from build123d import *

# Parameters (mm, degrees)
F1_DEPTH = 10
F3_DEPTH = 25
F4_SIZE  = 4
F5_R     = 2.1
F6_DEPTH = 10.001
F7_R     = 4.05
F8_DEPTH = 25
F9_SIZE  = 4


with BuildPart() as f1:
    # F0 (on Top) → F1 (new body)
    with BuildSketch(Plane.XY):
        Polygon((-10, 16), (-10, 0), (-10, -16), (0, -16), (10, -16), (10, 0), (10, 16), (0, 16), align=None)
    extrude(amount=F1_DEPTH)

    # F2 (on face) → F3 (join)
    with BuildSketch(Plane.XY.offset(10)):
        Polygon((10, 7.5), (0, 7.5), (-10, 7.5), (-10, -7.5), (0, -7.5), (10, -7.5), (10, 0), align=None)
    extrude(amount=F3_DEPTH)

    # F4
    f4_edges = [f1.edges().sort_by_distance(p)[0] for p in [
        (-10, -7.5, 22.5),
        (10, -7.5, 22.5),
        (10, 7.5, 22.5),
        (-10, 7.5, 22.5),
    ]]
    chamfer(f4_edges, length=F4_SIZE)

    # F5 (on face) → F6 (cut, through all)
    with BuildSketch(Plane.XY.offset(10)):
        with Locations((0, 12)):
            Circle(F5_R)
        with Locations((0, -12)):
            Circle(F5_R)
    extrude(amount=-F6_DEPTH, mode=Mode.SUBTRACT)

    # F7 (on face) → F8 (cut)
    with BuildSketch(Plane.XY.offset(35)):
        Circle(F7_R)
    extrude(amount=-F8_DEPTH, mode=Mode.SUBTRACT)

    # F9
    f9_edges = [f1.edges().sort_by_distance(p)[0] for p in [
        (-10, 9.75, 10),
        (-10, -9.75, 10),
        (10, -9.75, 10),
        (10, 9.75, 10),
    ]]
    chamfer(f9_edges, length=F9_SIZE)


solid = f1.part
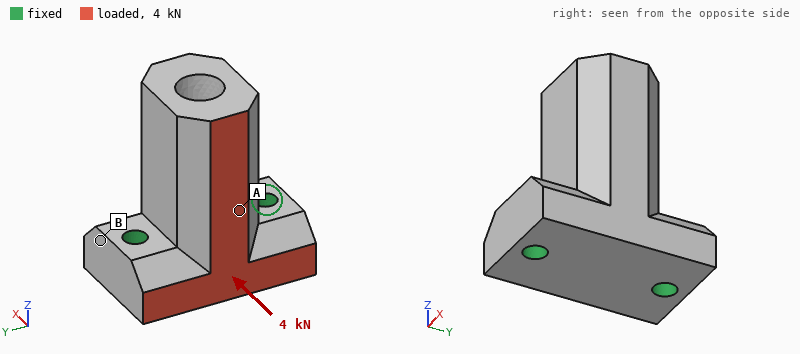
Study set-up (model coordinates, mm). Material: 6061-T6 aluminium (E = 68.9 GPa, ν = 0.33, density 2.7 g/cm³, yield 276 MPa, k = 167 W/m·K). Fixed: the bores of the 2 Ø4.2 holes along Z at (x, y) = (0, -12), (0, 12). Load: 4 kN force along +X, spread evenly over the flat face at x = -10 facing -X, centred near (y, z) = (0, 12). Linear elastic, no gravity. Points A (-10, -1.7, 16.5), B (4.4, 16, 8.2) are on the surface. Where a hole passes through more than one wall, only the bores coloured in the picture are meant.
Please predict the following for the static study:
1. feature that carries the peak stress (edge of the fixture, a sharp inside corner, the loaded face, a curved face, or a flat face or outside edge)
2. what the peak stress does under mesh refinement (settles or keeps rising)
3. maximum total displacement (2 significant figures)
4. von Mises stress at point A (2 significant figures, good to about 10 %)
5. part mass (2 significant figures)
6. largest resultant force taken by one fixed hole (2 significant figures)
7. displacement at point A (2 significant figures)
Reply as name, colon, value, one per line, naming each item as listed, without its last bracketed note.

feature that carries the peak stress: edge of the fixture
what the peak stress does under mesh refinement: keeps rising
maximum total displacement: 59 µm
von Mises stress at point A: 21 MPa
part mass: 30 g
largest resultant force taken by one fixed hole: 2.0 kN
displacement at point A: 27 µm
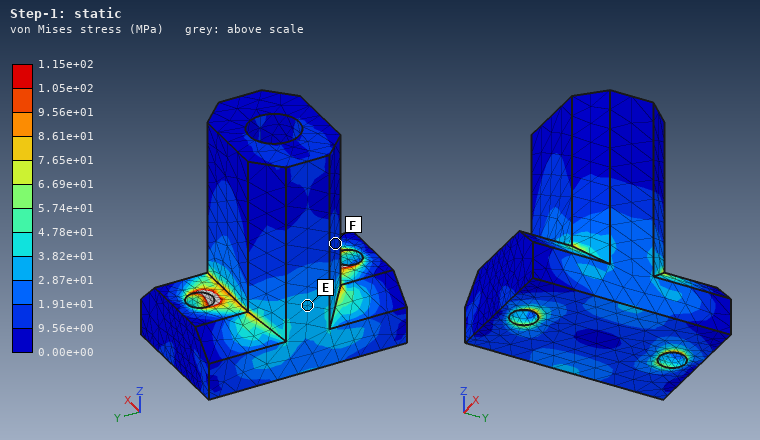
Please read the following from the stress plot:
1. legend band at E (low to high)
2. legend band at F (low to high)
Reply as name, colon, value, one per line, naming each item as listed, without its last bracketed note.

legend band at E: 2.87e+01 to 3.82e+01 MPa
legend band at F: 9.56e+00 to 1.91e+01 MPa
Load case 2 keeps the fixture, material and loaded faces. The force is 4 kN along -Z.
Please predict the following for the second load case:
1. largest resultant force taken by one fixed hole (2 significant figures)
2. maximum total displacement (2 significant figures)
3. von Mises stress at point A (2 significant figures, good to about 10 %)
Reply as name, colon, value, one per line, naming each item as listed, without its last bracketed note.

largest resultant force taken by one fixed hole: 2.0 kN
maximum total displacement: 58 µm
von Mises stress at point A: 27 MPa
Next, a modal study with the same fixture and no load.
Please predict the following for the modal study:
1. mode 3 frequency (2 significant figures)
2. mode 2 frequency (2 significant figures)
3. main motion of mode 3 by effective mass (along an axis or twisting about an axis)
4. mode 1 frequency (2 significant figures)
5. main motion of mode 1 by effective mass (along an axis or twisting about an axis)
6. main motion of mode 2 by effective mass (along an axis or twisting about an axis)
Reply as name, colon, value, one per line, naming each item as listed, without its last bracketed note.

mode 3 frequency: 26 kHz
mode 2 frequency: 12 kHz
main motion of mode 3 by effective mass: twisting about Z
mode 1 frequency: 8700 Hz
main motion of mode 1 by effective mass: along X
main motion of mode 2 by effective mass: along Y
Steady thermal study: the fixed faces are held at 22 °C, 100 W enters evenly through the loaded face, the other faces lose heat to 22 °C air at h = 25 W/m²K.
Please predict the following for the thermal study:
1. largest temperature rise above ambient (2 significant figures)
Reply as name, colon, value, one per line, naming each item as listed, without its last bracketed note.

largest temperature rise above ambient: 37 K
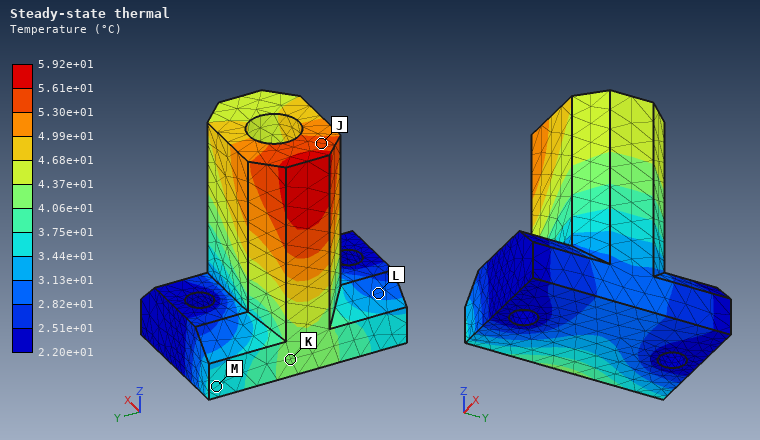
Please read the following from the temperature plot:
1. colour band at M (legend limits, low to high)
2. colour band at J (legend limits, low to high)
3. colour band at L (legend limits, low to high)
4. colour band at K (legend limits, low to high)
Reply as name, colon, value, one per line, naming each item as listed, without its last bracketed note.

colour band at M: 3.44e+01 to 3.75e+01 °C
colour band at J: 5.30e+01 to 5.61e+01 °C
colour band at L: 2.82e+01 to 3.13e+01 °C
colour band at K: 4.06e+01 to 4.37e+01 °C
